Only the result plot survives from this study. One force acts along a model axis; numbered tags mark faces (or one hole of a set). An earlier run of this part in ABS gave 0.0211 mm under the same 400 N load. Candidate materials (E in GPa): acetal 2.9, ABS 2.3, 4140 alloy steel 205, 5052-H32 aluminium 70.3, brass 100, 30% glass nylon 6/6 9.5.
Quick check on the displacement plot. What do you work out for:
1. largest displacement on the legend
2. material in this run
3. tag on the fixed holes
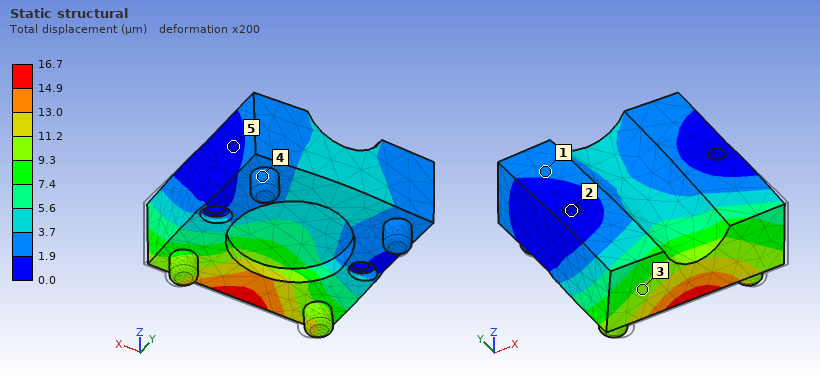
16.7 µm
acetal
2
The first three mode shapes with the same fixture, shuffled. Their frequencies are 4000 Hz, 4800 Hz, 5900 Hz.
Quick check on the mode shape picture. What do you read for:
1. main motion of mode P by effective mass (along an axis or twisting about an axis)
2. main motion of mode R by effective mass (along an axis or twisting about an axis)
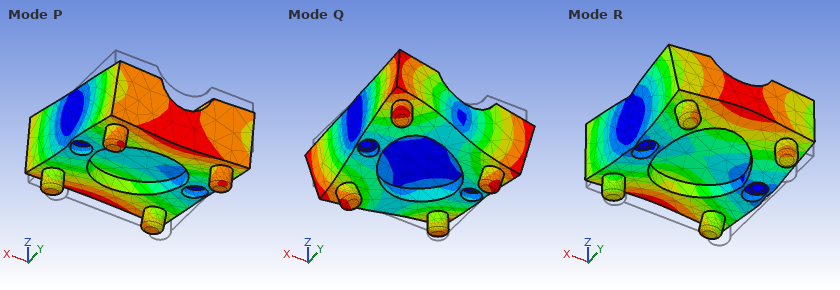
twisting about X
along Z
